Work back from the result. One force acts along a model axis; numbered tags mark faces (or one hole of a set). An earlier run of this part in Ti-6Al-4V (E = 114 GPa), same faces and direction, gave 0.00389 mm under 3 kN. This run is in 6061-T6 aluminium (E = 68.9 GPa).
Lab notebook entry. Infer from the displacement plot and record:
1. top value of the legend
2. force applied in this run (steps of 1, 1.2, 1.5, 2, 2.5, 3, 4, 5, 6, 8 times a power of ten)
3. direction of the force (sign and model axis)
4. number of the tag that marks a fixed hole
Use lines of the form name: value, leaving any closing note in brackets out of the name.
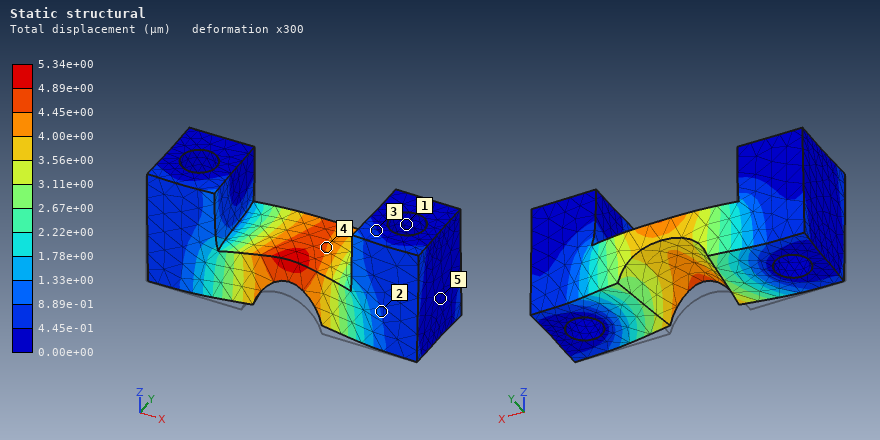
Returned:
top value of the legend: 5.34e+00 µm
force applied in this run: 2.5 kN
direction of the force: +Y
number of the tag that marks a fixed hole: 1
